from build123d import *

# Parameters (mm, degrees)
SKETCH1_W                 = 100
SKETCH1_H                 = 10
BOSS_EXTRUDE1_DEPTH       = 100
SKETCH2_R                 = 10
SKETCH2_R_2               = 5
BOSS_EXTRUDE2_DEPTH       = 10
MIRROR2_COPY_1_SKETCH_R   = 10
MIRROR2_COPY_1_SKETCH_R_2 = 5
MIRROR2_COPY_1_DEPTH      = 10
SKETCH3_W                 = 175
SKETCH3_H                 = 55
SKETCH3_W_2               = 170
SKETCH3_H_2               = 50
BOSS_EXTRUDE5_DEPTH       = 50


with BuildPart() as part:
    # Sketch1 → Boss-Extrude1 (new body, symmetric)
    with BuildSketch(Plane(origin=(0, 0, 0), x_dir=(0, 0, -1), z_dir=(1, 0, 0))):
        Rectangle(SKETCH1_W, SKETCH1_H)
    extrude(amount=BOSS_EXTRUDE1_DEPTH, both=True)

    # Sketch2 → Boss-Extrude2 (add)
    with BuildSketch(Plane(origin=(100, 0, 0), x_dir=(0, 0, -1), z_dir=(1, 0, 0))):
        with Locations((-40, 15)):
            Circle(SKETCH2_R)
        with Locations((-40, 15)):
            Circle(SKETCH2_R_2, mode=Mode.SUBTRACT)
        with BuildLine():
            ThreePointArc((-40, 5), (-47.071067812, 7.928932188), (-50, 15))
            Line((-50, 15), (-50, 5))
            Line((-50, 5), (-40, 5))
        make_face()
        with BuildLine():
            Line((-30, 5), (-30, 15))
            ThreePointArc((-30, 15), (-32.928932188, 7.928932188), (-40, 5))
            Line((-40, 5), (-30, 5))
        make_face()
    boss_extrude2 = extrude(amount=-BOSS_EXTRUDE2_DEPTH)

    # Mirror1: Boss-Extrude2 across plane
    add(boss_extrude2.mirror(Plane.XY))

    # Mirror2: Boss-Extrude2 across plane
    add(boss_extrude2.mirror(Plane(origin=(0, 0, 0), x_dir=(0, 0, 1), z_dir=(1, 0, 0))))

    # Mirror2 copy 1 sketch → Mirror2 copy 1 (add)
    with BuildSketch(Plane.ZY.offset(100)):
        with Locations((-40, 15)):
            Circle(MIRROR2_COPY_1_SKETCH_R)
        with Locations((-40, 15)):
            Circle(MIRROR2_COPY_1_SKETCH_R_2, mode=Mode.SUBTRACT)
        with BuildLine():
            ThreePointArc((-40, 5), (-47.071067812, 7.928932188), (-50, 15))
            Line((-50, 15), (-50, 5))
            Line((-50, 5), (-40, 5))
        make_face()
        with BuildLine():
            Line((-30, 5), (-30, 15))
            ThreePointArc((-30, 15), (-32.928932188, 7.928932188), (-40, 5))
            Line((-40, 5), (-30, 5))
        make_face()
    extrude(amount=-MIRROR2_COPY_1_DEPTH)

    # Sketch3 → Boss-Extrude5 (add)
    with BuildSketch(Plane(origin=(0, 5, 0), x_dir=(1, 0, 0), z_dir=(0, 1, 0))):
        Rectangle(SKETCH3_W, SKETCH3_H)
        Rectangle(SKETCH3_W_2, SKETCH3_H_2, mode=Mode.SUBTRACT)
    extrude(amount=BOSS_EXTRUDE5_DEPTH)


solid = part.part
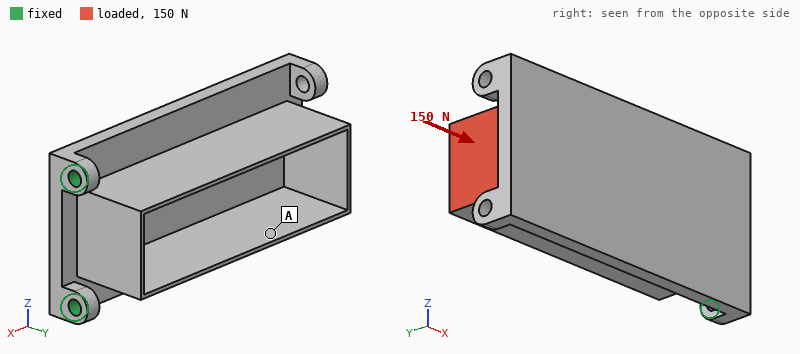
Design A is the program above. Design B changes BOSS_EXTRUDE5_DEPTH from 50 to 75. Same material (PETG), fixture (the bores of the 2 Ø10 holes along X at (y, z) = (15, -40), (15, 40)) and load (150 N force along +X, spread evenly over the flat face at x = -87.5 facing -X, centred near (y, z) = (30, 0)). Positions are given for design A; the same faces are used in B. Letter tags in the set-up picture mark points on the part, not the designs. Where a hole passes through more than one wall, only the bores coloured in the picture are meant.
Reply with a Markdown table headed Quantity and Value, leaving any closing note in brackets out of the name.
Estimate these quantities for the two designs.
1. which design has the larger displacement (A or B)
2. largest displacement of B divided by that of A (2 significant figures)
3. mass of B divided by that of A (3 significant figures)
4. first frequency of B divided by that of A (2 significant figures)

| Quantity | Value |
|---|---|
| which design has the larger displacement | B |
| largest displacement of B divided by that of A | 1.4 |
| mass of B divided by that of A | 1.11 |
| first frequency of B divided by that of A | 0.94 |
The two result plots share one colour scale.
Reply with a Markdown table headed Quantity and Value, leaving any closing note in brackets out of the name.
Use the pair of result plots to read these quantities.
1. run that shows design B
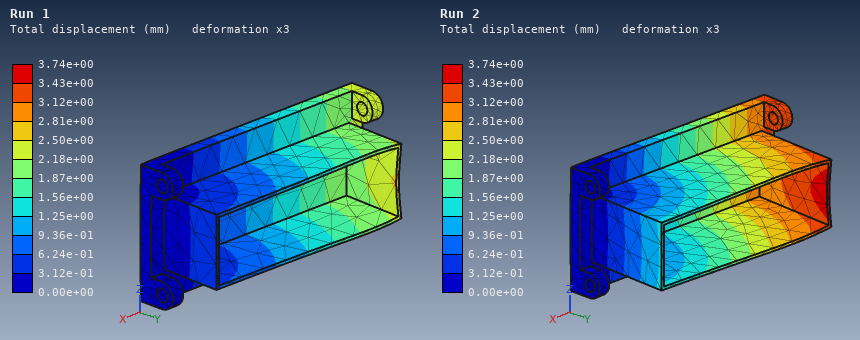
| Quantity | Value |
|---|---|
| run that shows design B | Run 2 |
